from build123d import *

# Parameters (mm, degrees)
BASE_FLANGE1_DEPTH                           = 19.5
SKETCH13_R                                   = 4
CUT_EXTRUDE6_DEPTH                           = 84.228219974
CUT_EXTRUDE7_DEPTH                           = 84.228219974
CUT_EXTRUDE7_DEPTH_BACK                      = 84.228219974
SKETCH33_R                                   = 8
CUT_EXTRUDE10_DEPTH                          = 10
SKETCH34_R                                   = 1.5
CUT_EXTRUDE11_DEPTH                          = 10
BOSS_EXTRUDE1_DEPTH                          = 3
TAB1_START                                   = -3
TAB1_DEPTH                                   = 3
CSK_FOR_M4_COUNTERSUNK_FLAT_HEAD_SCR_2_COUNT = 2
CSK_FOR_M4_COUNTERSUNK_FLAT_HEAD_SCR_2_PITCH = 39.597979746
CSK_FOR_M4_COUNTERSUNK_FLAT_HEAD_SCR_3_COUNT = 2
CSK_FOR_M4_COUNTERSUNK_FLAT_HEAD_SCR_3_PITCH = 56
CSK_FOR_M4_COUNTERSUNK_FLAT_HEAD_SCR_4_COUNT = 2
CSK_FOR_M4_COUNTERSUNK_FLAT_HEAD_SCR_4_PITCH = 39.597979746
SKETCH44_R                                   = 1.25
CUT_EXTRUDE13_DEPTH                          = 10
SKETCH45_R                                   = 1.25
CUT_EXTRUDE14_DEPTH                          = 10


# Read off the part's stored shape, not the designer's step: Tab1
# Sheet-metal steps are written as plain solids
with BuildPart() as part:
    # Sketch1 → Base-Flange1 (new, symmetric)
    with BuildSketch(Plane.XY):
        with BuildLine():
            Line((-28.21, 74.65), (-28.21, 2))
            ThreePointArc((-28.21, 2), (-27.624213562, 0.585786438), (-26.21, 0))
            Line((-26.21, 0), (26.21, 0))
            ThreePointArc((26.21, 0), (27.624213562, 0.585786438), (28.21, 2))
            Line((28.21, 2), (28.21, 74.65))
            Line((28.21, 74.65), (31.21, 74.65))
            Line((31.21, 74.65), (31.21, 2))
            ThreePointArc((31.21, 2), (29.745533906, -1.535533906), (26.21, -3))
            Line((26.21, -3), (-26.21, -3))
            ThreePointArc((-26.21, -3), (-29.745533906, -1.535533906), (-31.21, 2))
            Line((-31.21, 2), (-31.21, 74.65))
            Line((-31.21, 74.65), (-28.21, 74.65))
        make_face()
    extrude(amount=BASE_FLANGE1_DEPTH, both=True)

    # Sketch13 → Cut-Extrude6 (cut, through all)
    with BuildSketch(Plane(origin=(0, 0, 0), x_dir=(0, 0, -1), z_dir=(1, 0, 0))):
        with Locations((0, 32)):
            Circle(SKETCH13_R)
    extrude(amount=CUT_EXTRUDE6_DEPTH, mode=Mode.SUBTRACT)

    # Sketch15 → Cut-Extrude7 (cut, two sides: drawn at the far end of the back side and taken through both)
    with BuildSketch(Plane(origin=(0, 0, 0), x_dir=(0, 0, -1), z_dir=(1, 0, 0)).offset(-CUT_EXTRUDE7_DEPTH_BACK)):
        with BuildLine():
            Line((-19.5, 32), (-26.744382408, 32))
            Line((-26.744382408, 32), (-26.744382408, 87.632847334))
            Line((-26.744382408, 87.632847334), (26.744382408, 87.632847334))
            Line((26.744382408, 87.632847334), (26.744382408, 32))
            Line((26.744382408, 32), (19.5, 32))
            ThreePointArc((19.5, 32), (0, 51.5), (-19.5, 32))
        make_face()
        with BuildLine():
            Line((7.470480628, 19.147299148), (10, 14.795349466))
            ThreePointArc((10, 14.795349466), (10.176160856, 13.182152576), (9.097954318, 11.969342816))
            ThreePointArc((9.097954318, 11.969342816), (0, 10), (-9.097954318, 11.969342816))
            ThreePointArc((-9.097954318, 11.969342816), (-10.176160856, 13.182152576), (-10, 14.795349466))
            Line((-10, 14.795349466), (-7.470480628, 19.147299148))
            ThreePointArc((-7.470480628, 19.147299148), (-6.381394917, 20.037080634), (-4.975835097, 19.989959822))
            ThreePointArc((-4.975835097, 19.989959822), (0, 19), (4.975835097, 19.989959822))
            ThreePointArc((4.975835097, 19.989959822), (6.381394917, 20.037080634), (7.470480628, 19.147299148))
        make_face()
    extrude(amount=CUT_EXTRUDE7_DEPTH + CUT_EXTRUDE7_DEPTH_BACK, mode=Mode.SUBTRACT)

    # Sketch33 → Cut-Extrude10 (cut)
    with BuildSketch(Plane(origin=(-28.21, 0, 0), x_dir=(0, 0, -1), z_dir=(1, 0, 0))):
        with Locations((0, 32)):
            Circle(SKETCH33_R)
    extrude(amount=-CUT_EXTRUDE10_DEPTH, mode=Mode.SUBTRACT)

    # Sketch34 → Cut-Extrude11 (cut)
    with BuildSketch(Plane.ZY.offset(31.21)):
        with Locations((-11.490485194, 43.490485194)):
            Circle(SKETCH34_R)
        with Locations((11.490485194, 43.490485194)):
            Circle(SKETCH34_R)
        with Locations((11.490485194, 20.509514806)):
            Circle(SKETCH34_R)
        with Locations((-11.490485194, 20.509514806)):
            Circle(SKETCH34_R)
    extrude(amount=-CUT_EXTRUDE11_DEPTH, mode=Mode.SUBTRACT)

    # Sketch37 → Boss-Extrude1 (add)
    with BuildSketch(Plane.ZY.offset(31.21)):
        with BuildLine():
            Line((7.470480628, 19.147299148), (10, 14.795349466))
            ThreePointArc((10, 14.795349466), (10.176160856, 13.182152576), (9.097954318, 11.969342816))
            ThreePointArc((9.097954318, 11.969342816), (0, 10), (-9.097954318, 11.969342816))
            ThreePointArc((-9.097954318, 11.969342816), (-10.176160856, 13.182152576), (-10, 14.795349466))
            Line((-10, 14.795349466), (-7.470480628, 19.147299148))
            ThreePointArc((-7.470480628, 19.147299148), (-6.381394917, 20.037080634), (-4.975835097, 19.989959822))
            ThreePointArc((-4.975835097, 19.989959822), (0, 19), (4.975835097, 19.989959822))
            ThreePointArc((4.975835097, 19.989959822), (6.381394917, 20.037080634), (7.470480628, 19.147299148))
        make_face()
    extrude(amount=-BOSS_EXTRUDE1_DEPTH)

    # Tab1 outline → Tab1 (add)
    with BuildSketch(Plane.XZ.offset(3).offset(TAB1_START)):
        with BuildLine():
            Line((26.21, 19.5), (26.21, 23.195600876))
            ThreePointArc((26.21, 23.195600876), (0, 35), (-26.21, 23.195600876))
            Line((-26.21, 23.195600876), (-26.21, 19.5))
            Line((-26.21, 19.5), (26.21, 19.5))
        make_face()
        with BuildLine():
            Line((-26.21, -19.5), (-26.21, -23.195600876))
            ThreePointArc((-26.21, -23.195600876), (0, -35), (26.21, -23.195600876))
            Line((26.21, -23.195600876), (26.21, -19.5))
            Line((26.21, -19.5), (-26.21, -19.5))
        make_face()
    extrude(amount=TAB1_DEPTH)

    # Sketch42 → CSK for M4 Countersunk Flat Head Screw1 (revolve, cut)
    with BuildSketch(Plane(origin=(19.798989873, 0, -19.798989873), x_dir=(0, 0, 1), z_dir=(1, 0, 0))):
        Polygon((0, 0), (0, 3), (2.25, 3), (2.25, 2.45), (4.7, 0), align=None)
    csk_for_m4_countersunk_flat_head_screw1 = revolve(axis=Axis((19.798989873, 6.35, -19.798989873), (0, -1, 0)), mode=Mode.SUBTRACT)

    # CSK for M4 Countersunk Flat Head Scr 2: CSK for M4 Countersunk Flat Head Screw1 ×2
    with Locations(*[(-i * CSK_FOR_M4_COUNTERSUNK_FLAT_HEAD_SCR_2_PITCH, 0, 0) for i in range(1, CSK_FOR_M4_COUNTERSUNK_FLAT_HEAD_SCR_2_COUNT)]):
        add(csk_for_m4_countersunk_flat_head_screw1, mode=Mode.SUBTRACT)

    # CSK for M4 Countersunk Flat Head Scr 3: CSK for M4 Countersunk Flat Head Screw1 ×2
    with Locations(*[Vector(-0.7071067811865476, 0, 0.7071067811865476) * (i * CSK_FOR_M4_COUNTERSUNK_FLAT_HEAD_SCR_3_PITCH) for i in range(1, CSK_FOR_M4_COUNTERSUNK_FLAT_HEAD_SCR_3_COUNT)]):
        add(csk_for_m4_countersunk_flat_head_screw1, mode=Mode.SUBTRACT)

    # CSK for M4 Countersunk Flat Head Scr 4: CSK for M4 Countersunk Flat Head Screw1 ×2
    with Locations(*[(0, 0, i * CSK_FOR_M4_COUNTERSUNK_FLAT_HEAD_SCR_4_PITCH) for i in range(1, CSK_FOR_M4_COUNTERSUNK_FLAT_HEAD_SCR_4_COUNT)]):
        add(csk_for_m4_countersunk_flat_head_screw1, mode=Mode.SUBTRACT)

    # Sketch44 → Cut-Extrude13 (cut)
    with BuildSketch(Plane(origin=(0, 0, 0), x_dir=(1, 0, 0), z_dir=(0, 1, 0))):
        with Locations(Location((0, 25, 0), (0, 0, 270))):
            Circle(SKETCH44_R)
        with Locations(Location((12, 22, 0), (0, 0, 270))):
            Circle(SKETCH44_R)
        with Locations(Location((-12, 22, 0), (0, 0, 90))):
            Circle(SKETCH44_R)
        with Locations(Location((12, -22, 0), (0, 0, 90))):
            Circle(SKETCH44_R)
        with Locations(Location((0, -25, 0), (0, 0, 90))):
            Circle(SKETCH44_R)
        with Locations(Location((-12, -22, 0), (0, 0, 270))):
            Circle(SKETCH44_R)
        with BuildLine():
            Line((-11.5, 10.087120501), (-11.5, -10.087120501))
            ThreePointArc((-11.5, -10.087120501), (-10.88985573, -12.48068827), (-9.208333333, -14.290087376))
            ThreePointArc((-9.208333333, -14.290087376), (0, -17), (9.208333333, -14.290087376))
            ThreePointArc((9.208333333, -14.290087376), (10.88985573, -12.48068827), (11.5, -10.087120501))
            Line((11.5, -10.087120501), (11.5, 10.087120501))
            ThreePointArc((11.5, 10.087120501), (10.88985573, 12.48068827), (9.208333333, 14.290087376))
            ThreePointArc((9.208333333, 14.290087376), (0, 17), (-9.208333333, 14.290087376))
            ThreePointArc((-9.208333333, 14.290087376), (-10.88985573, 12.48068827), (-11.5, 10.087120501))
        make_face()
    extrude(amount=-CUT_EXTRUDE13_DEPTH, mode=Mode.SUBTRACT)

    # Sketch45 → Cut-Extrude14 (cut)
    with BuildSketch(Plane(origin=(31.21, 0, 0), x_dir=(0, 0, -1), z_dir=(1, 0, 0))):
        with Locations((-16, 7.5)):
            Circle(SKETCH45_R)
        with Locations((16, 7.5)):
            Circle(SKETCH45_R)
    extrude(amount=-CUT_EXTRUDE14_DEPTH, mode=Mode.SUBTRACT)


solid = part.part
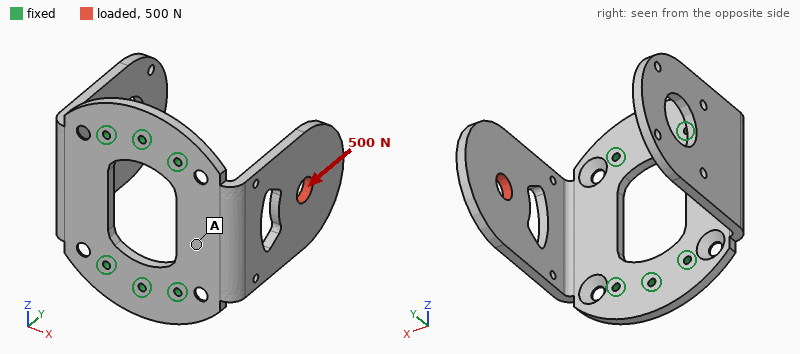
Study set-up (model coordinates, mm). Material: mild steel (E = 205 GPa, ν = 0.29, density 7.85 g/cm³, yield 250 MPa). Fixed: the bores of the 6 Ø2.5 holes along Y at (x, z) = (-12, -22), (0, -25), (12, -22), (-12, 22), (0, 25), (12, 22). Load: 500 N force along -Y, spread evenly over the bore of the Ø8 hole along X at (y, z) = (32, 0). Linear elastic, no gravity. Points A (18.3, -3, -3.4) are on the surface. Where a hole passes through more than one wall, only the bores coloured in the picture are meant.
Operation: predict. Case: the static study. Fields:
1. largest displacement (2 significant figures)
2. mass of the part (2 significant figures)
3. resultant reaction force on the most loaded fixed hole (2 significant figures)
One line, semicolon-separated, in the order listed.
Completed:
0.33 mm; 140 g; 400 N
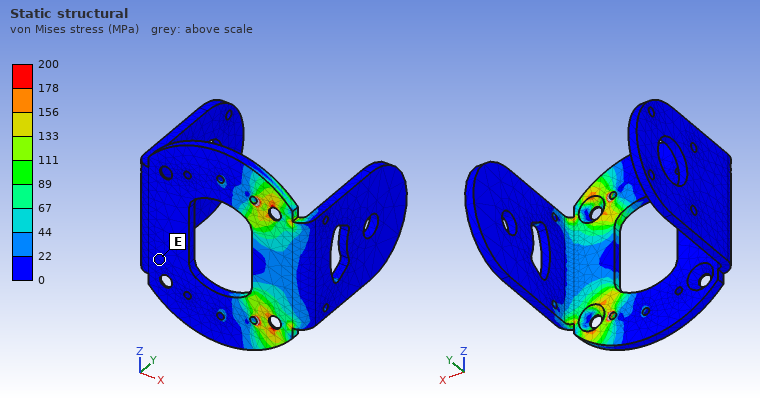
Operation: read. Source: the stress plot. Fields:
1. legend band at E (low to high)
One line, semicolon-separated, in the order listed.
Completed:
0 to 22 MPa
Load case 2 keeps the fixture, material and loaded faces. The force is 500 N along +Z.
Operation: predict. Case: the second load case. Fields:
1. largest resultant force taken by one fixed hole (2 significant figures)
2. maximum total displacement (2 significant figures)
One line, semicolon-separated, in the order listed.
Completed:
610 N; 0.19 mm
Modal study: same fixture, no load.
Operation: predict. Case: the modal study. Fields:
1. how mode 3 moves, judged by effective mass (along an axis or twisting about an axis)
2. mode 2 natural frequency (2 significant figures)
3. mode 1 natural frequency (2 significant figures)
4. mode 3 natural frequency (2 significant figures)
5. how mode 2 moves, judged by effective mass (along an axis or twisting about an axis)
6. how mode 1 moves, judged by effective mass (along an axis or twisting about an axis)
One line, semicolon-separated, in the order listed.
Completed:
along Z; 660 Hz; 580 Hz; 1700 Hz; along X; along X
